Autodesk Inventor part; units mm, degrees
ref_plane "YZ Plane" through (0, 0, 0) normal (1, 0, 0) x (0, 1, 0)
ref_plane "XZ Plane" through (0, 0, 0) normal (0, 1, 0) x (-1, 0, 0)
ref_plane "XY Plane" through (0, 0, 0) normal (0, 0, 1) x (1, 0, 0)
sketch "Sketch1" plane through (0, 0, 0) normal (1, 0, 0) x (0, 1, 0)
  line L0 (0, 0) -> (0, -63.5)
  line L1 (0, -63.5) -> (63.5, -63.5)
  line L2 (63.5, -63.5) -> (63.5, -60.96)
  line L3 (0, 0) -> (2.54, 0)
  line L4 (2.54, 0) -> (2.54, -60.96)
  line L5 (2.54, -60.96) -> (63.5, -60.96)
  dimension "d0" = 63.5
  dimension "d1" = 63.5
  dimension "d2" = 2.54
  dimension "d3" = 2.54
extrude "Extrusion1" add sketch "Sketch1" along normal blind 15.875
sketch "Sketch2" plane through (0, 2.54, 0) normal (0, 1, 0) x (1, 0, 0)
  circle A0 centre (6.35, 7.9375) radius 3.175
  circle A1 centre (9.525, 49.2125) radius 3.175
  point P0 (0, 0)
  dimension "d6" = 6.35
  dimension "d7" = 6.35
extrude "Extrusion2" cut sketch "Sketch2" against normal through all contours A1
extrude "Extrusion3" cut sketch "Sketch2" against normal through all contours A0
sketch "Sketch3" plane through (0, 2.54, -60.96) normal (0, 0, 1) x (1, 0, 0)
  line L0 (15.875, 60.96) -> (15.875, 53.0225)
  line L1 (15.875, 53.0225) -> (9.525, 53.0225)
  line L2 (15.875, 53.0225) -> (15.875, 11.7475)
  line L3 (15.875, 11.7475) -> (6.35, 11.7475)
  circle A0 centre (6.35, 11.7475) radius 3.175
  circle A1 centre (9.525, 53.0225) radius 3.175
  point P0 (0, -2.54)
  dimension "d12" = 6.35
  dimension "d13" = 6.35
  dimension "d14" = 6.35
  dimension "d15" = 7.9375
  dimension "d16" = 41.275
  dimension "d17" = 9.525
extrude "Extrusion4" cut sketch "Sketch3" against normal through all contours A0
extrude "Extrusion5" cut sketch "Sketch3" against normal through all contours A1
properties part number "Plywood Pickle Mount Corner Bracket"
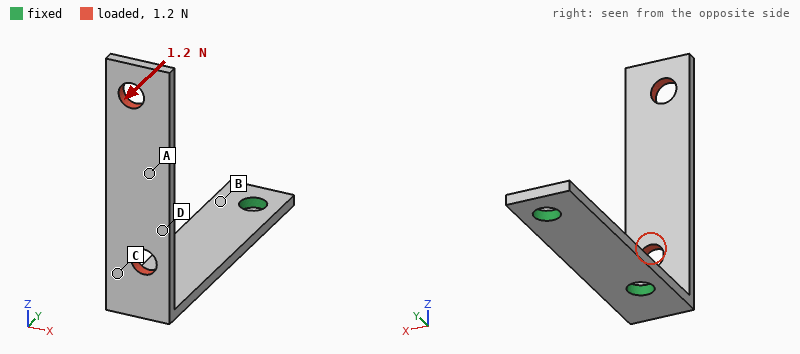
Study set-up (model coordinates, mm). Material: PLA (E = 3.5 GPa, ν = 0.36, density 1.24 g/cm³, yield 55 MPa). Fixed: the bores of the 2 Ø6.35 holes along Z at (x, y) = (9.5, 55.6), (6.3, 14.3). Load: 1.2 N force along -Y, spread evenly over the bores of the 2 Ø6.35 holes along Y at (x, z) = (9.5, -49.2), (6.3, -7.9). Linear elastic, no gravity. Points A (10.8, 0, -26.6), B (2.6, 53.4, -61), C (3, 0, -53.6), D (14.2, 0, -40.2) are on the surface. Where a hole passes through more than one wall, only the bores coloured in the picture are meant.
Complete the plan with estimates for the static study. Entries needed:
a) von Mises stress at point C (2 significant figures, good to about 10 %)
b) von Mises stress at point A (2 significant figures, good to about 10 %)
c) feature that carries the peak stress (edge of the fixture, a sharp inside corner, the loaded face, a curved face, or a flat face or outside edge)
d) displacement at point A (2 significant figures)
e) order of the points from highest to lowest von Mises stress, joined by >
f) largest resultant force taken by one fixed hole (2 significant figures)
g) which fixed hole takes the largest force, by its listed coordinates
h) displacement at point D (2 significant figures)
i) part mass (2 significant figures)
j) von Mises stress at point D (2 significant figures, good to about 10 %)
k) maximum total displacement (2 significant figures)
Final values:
2.1 MPa
0.66 MPa
a flat face or outside edge
0.44 mm
C > D > A > B
1.2 N
(6.3, 14.3)
0.23 mm
5.8 g
1.1 MPa
0.93 mm
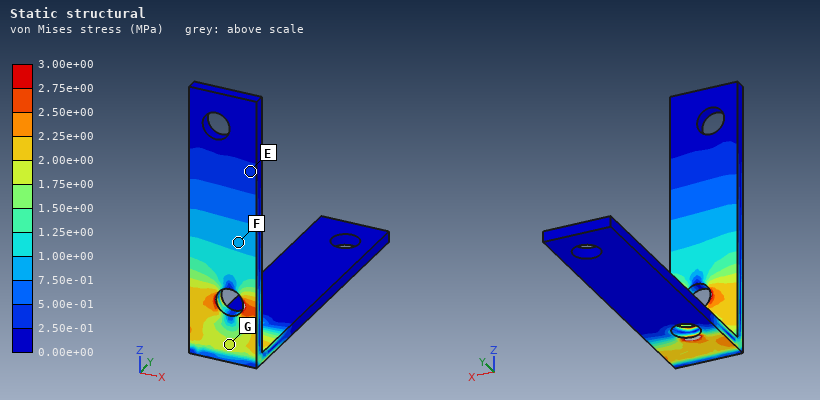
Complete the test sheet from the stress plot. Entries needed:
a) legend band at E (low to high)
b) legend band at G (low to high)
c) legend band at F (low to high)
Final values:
2.50e-01 to 5.00e-01 MPa
1.75e+00 to 2.00e+00 MPa
7.50e-01 to 1.00e+00 MPa
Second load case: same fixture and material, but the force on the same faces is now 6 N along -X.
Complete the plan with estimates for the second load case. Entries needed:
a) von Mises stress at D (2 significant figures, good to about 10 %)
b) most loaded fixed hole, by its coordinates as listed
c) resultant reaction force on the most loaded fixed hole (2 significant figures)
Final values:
0.76 MPa
(6.3, 14.3)
6.6 N
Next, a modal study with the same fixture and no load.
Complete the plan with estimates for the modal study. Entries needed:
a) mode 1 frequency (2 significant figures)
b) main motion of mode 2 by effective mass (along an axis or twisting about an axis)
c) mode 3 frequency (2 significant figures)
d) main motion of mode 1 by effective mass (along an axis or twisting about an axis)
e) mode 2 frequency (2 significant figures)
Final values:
140 Hz
along X
900 Hz
along Y
290 Hz
